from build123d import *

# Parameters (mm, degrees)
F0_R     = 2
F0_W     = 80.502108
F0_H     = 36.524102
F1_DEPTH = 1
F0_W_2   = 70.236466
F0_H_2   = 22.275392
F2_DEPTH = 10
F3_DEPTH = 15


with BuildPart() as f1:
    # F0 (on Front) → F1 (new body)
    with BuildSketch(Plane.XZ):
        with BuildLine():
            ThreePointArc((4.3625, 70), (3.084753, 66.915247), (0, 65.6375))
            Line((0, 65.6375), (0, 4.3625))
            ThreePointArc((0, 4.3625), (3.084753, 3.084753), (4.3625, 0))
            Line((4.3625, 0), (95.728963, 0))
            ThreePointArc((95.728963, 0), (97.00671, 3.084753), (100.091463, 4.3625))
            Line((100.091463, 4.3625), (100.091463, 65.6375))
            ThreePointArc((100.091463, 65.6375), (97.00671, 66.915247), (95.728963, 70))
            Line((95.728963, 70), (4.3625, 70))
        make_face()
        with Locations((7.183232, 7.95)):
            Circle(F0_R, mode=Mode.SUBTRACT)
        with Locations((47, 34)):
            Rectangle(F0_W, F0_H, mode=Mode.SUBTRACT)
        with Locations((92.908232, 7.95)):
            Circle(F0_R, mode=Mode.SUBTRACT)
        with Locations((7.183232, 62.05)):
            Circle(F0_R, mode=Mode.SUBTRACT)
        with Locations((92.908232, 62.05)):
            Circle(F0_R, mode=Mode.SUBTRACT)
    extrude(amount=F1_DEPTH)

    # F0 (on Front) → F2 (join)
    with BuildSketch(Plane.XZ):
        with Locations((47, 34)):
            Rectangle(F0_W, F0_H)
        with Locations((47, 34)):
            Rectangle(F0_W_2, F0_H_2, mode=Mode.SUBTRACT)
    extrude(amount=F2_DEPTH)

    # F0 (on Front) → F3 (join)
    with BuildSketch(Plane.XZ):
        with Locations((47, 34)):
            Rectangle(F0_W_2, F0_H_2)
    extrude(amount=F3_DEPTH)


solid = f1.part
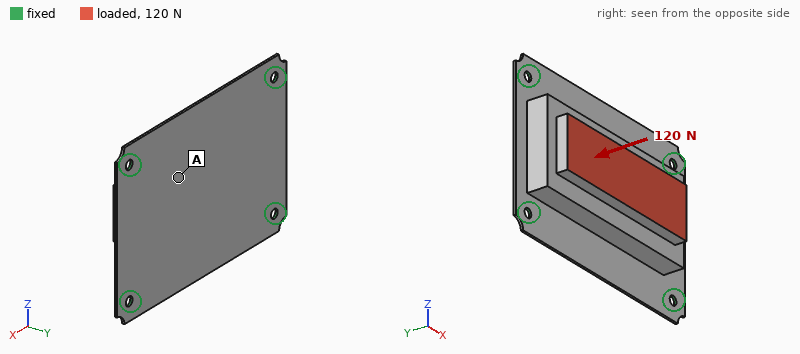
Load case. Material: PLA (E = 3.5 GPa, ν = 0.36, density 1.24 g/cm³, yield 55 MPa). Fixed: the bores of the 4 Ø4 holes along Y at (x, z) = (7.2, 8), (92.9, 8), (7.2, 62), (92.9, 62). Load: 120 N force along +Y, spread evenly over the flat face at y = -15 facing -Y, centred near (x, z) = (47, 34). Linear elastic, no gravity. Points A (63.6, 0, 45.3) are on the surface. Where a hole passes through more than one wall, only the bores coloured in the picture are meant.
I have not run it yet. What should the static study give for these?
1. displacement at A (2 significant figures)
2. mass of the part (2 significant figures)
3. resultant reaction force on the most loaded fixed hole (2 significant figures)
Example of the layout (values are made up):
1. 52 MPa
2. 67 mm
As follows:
1. 0.56 mm
2. 51 g
3. 43 N
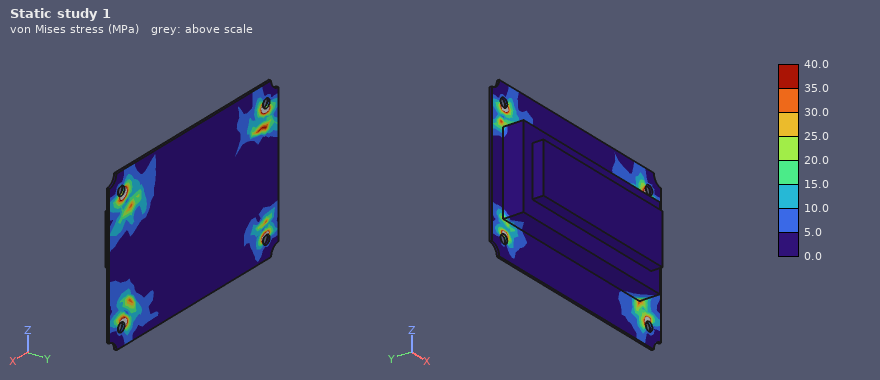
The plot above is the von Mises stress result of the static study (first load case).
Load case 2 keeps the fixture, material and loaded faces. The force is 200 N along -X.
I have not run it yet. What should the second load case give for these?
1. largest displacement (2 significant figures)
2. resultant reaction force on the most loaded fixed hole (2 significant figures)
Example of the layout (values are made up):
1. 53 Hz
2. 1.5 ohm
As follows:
1. 0.39 mm
2. 65 N
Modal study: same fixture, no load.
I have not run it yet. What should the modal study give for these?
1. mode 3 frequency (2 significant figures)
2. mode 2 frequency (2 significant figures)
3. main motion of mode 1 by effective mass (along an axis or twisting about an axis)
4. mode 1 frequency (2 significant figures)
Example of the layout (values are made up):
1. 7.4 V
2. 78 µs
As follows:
1. 680 Hz
2. 620 Hz
3. along Y
4. 360 Hz
